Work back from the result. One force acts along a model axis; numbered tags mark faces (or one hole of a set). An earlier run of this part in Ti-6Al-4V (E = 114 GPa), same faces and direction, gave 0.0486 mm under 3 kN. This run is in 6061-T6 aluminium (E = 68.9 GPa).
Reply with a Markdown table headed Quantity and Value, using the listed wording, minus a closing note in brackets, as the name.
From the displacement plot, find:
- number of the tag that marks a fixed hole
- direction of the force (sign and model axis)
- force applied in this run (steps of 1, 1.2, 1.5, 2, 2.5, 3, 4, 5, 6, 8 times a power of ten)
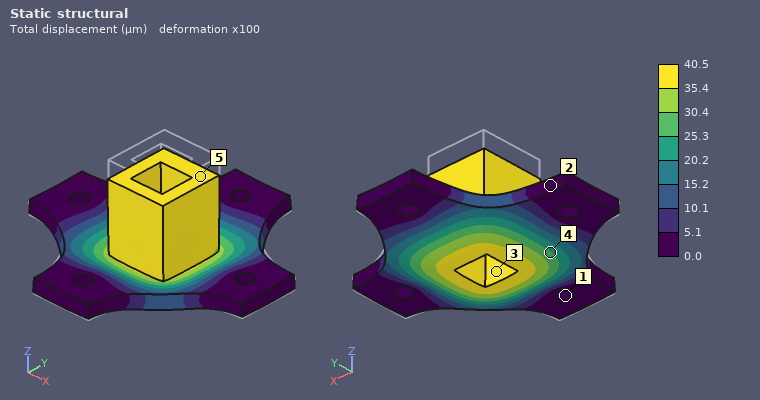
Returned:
| Quantity | Value |
|---|---|
| number of the tag that marks a fixed hole | 1 |
| direction of the force | -Z |
| force applied in this run | 1.5 kN |
